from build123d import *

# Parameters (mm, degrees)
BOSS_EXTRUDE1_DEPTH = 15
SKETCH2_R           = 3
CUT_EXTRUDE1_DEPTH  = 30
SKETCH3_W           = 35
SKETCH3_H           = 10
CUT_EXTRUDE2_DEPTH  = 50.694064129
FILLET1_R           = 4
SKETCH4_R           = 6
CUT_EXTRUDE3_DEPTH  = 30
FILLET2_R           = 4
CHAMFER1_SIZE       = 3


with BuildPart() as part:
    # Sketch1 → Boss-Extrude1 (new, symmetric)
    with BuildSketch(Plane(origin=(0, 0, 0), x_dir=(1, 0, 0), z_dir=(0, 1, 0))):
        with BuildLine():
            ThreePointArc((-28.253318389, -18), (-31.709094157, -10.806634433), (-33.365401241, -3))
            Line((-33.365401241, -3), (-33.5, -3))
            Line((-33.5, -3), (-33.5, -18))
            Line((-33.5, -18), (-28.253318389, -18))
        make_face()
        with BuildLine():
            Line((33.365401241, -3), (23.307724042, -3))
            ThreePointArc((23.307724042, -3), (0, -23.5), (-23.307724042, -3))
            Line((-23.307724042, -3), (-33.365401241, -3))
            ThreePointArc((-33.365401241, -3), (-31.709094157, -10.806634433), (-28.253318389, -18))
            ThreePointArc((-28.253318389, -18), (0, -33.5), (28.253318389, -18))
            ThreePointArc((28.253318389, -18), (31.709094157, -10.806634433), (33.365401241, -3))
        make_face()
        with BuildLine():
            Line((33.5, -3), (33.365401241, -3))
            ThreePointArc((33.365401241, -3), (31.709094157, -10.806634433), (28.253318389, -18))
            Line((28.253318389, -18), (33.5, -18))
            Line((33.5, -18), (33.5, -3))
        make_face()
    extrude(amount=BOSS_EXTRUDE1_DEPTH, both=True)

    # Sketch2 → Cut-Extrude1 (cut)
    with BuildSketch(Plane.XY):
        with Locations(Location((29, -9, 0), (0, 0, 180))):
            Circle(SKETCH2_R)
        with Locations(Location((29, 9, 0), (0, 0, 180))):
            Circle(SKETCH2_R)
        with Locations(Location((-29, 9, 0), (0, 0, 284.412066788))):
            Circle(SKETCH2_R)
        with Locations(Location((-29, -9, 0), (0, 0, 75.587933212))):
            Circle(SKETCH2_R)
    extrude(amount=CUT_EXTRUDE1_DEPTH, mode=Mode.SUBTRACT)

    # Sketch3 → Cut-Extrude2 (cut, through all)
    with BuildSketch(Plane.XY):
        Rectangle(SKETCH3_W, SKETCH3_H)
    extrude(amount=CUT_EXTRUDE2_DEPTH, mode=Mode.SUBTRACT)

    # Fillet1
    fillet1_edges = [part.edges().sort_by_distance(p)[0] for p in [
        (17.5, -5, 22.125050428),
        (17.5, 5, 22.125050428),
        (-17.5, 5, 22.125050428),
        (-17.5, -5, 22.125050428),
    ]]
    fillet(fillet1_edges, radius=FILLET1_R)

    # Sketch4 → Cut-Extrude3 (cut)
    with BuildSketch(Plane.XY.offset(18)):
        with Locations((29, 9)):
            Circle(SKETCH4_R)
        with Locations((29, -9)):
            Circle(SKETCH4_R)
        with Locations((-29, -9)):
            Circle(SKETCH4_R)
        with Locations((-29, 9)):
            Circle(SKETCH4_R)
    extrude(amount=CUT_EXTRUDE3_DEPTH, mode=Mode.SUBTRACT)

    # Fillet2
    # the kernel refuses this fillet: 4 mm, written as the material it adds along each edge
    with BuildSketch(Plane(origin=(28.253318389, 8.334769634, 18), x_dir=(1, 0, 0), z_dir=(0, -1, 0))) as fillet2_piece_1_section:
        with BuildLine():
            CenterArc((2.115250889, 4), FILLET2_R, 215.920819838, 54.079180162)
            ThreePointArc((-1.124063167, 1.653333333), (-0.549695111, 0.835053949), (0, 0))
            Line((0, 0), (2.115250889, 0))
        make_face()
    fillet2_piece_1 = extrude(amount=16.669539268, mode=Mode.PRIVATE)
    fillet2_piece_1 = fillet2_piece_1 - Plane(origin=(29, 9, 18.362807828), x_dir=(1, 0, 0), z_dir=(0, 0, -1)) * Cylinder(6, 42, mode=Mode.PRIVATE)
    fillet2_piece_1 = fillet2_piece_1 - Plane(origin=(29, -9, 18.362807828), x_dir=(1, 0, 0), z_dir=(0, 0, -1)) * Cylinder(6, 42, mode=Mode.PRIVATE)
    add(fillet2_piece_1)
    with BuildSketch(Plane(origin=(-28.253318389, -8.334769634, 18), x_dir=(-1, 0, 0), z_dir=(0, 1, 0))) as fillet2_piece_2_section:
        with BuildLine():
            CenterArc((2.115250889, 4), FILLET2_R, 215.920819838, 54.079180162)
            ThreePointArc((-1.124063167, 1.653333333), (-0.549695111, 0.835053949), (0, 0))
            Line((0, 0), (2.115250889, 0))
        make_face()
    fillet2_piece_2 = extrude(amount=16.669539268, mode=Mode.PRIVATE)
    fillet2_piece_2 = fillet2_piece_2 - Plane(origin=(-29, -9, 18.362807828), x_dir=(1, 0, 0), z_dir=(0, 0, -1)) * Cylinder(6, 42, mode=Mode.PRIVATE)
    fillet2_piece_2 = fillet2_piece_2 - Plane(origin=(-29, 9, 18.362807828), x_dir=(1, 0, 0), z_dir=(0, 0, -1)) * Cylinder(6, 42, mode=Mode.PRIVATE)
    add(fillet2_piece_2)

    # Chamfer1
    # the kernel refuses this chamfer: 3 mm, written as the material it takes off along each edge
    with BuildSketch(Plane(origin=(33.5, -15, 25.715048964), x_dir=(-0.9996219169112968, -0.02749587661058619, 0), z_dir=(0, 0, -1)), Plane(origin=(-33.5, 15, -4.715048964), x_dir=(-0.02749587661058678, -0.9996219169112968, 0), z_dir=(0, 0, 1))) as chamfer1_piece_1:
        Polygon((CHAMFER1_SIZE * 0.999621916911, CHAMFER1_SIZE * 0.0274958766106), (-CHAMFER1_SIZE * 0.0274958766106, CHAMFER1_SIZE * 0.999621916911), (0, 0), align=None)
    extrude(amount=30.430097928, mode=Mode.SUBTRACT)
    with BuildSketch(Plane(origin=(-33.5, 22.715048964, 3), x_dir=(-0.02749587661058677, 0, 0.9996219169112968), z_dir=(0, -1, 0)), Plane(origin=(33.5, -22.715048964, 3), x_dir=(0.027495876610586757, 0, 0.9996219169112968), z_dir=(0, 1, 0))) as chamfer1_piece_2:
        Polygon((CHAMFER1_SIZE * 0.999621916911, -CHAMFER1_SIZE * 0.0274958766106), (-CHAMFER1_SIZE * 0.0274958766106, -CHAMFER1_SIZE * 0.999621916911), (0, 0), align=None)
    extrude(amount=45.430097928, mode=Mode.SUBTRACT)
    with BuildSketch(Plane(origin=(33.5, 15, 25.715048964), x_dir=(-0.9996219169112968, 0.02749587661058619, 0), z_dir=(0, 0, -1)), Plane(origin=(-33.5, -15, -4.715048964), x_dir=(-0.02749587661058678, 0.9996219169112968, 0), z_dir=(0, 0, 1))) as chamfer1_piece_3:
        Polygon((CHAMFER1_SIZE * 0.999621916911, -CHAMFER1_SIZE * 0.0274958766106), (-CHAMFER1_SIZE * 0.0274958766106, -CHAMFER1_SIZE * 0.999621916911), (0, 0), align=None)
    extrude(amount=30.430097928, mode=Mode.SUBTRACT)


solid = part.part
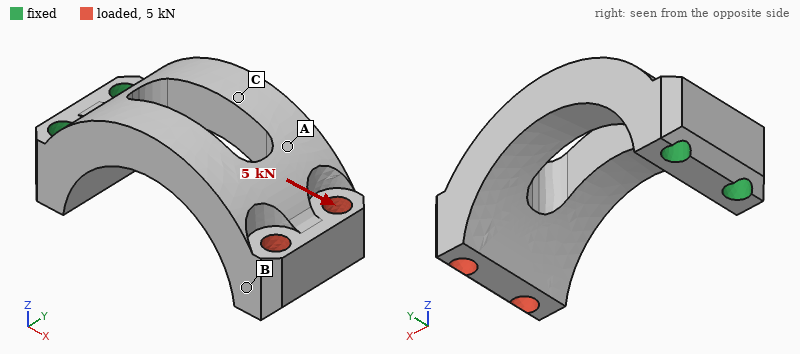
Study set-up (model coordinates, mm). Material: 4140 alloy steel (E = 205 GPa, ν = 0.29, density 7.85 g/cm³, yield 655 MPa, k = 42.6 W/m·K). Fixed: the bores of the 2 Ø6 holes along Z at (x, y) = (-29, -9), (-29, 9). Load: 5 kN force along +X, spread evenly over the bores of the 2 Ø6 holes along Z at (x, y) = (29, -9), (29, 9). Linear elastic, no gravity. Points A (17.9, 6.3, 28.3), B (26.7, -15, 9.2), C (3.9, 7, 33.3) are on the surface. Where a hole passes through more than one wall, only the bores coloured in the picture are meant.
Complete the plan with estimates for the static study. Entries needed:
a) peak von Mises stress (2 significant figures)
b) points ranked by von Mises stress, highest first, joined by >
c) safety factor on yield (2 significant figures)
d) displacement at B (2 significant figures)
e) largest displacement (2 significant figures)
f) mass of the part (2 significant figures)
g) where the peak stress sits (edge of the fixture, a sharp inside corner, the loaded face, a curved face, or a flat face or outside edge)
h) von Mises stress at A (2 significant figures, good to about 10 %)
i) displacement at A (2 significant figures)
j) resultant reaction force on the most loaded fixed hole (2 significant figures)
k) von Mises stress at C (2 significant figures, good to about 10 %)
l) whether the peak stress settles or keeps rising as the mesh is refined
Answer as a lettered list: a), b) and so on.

a) 330 MPa
b) C > A > B
c) 2.0
d) 0.35 mm
e) 0.44 mm
f) 160 g
g) a curved face
h) 140 MPa
i) 0.21 mm
j) 2.5 kN
k) 210 MPa
l) settles
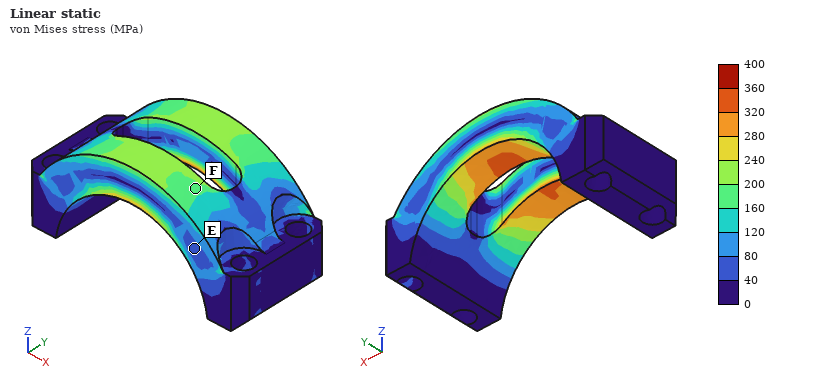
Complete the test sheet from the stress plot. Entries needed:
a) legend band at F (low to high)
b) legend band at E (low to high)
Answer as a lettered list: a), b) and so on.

a) 160 to 200 MPa
b) 40 to 80 MPa
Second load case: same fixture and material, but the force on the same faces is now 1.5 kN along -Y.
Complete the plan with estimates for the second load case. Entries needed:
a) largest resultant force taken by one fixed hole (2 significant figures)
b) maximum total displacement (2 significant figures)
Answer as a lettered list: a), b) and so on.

a) 3.8 kN
b) 0.21 mm
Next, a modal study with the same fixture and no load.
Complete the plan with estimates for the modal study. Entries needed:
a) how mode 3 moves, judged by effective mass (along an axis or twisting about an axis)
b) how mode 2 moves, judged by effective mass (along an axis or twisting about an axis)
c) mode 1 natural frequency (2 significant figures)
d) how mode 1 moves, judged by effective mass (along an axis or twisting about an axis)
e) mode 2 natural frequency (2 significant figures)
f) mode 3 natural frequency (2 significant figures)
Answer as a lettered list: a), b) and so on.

a) along X
b) along Y
c) 1500 Hz
d) along Z
e) 2100 Hz
f) 5300 Hz
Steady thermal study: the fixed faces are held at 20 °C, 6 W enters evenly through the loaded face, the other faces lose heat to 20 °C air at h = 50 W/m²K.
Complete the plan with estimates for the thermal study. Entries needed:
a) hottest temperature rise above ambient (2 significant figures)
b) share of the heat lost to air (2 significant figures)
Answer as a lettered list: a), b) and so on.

a) 23 K
b) 61 %
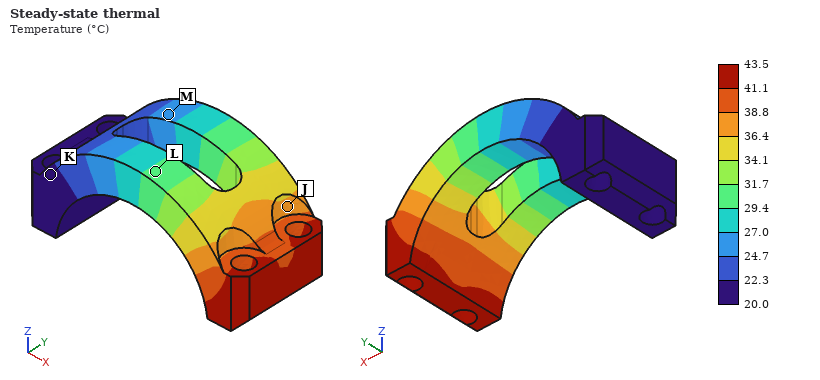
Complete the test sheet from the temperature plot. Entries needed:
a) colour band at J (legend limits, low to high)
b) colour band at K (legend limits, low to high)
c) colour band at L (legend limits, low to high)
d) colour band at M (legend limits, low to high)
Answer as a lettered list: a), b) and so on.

a) 36.4 to 38.8 °C
b) 20.0 to 22.3 °C
c) 29.4 to 31.7 °C
d) 24.7 to 27.0 °C
